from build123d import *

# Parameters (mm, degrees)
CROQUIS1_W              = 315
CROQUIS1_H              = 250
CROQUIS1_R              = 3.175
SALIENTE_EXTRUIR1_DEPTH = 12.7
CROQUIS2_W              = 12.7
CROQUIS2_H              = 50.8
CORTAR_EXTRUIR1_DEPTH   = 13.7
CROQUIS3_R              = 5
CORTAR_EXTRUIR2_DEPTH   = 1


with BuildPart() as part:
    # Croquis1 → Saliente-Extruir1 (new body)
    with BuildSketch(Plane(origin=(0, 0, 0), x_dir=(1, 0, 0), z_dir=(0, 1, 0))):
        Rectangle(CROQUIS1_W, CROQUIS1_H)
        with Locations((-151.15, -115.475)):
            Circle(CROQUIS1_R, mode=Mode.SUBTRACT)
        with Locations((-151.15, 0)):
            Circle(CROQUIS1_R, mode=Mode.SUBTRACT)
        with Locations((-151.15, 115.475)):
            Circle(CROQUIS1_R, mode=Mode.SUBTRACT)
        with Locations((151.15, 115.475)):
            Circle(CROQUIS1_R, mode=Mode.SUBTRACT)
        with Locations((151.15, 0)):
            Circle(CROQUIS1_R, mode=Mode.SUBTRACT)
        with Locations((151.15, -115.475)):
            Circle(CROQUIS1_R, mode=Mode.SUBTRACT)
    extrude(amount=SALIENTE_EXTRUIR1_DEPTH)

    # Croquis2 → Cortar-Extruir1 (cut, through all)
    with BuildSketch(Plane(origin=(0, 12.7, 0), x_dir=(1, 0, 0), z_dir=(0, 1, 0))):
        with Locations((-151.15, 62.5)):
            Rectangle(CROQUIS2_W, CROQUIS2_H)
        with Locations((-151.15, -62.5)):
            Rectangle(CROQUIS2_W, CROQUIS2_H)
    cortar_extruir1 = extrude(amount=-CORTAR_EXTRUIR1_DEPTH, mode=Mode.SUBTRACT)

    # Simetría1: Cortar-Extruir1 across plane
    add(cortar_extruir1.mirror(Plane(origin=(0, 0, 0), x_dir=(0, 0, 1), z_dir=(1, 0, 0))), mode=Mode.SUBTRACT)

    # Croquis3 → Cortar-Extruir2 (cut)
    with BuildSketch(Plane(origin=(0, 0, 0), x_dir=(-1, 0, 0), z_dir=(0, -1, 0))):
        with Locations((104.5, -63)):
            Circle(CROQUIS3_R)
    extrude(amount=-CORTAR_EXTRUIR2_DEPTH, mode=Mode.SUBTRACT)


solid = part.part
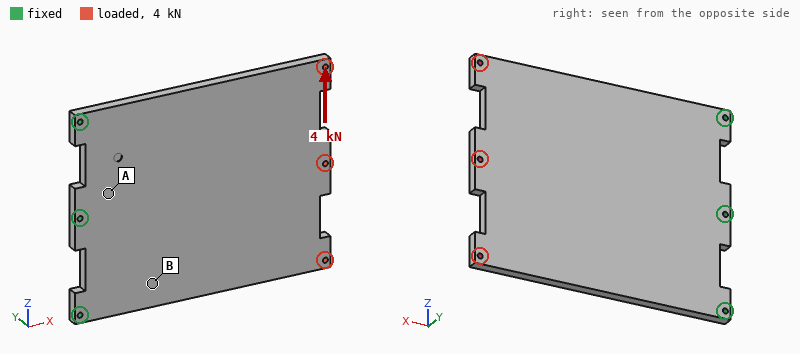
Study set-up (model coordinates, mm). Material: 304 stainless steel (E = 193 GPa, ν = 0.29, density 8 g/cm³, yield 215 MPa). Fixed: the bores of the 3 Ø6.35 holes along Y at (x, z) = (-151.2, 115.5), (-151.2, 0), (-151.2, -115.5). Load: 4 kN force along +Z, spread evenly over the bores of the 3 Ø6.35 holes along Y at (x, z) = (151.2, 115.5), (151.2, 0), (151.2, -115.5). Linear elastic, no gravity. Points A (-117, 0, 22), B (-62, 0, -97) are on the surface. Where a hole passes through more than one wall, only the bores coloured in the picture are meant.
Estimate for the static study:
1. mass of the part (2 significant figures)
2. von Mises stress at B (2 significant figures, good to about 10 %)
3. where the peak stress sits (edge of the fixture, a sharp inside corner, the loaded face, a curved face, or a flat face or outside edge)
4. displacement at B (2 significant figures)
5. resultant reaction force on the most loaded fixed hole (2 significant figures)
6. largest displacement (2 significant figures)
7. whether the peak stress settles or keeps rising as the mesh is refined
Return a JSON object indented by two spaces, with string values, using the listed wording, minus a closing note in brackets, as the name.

{
  "mass of the part": "7.7 kg",
  "von Mises stress at B": "5.6 MPa",
  "where the peak stress sits": "edge of the fixture",
  "displacement at B": "6.0 µm",
  "resultant reaction force on the most loaded fixed hole": "5.6 kN",
  "largest displacement": "27 µm",
  "whether the peak stress settles or keeps rising as the mesh is refined": "keeps rising"
}
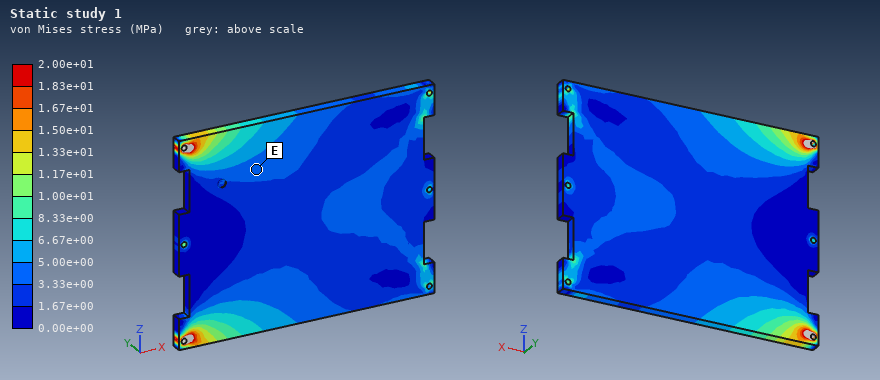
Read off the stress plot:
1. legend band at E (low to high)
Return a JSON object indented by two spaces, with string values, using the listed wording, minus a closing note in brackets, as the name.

{
  "legend band at E": "3.33e+00 to 5.00e+00 MPa"
}
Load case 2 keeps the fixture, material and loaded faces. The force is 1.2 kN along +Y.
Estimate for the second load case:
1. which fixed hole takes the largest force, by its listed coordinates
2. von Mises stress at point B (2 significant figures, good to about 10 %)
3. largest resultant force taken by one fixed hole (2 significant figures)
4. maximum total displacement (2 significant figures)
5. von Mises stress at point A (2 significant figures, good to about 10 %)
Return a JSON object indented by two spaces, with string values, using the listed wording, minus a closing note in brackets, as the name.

{
  "which fixed hole takes the largest force, by its listed coordinates": "(-151.2, 0)",
  "von Mises stress at point B": "39 MPa",
  "largest resultant force taken by one fixed hole": "1.1 kN",
  "maximum total displacement": "1.9 mm",
  "von Mises stress at point A": "45 MPa"
}
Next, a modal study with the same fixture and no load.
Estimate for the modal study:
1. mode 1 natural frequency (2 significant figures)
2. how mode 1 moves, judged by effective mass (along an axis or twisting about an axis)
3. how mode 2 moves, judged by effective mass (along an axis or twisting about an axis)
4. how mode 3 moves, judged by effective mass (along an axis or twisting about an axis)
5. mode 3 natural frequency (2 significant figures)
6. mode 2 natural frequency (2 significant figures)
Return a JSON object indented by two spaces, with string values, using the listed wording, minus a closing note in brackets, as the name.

{
  "mode 1 natural frequency": "91 Hz",
  "how mode 1 moves, judged by effective mass": "along Y",
  "how mode 2 moves, judged by effective mass": "twisting about X",
  "how mode 3 moves, judged by effective mass": "along Y",
  "mode 3 natural frequency": "610 Hz",
  "mode 2 natural frequency": "300 Hz"
}
